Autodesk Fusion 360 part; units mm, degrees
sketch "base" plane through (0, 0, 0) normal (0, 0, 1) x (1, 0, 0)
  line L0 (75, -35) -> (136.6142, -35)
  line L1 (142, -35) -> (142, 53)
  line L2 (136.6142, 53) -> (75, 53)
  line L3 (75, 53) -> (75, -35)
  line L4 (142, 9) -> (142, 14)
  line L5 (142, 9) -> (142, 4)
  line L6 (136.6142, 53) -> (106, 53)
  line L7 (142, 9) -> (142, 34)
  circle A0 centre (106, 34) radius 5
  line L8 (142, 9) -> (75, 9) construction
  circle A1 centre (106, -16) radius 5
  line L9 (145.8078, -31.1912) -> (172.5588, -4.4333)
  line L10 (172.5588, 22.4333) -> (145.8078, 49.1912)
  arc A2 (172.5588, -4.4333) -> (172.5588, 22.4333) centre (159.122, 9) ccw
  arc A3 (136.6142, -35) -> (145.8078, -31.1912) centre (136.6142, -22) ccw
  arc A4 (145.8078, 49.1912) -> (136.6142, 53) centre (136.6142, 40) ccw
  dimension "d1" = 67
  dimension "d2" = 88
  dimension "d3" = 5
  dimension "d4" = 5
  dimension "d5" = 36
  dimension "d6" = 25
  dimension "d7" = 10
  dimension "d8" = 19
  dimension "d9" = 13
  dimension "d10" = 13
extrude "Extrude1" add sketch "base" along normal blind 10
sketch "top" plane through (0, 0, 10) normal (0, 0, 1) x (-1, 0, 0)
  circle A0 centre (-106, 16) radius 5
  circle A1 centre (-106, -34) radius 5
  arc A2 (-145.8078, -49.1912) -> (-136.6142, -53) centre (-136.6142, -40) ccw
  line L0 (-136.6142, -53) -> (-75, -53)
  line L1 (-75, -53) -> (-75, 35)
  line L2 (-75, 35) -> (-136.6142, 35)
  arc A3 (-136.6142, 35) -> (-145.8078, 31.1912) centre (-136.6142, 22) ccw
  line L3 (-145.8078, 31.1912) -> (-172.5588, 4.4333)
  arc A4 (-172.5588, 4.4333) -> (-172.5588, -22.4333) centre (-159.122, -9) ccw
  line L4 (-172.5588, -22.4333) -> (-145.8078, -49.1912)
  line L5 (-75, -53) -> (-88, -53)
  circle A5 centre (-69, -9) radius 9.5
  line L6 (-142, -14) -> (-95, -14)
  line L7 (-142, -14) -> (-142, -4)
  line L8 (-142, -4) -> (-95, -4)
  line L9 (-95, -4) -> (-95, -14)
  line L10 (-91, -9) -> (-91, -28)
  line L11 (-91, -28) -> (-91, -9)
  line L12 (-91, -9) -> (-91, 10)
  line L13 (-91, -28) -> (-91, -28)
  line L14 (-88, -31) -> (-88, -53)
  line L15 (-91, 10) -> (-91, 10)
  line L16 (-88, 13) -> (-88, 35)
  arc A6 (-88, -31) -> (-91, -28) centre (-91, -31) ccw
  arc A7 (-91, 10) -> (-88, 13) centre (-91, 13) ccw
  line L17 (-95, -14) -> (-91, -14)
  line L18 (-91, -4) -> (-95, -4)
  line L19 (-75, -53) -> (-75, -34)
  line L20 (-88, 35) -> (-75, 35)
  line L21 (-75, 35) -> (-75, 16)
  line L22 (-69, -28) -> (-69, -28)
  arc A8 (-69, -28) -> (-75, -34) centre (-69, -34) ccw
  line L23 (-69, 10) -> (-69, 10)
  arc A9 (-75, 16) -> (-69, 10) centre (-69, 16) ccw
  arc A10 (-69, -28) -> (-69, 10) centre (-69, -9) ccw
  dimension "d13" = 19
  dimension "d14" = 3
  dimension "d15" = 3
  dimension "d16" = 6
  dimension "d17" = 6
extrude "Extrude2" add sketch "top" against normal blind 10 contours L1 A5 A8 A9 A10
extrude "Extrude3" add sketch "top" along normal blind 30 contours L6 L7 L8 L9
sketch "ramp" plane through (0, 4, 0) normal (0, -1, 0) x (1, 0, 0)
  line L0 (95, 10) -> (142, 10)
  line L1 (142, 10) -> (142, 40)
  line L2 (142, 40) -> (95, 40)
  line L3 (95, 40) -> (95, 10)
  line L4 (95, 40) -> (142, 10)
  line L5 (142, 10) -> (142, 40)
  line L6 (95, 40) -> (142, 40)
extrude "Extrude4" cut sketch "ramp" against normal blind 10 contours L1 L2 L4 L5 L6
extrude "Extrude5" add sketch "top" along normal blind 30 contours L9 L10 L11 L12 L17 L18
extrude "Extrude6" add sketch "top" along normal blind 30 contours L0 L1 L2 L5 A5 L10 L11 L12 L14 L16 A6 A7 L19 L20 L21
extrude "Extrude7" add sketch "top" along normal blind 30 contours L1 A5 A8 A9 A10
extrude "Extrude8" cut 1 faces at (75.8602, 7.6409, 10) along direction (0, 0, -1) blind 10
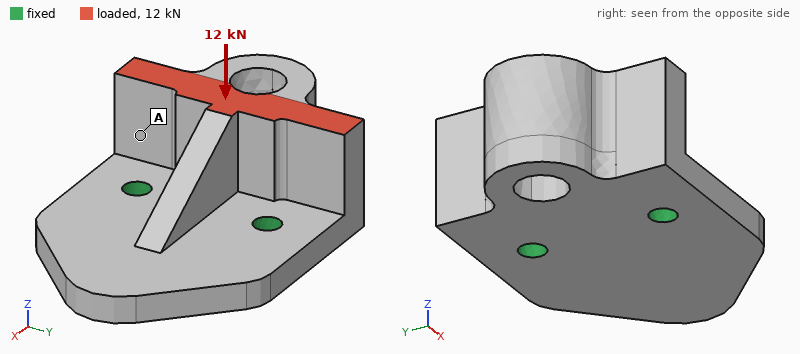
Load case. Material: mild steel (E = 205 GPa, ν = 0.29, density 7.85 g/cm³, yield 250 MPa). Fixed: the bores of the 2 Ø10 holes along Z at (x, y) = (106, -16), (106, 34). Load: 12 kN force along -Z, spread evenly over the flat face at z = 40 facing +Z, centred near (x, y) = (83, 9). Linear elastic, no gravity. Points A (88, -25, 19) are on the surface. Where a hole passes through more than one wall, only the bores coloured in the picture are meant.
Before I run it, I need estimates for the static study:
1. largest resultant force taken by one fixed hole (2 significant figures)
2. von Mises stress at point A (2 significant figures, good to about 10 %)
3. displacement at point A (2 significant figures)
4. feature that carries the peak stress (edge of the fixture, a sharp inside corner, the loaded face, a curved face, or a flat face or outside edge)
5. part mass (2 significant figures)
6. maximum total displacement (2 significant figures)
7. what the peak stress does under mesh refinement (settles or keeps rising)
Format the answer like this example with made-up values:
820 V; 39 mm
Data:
6.1 kN; 22 MPa; 28 µm; edge of the fixture; 1.1 kg; 78 µm; keeps rising
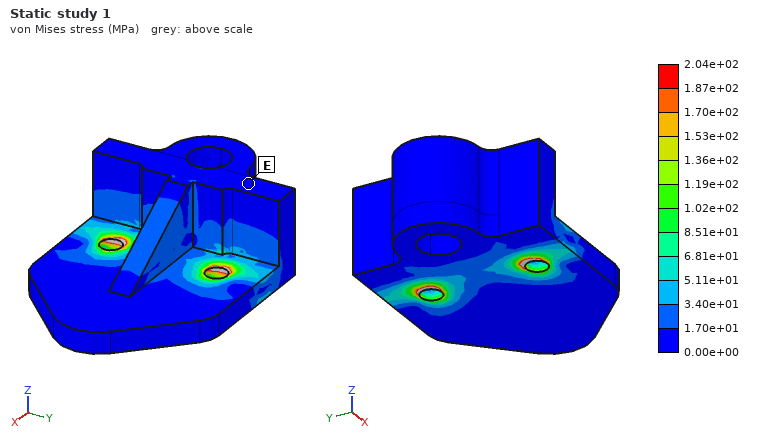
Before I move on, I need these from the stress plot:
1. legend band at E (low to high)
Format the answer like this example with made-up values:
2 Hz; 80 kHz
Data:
0.00e+00 to 1.70e+01 MPa
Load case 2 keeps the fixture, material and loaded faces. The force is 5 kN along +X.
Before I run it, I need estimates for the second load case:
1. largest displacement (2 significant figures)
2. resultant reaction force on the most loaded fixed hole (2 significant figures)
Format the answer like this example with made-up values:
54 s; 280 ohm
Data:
64 µm; 2.6 kN
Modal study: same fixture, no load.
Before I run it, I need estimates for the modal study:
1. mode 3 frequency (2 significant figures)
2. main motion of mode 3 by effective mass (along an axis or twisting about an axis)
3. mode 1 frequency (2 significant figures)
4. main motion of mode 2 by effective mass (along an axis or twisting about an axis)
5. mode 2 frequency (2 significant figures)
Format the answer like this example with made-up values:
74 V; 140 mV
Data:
5500 Hz; along Y; 2100 Hz; along Z; 3700 Hz
